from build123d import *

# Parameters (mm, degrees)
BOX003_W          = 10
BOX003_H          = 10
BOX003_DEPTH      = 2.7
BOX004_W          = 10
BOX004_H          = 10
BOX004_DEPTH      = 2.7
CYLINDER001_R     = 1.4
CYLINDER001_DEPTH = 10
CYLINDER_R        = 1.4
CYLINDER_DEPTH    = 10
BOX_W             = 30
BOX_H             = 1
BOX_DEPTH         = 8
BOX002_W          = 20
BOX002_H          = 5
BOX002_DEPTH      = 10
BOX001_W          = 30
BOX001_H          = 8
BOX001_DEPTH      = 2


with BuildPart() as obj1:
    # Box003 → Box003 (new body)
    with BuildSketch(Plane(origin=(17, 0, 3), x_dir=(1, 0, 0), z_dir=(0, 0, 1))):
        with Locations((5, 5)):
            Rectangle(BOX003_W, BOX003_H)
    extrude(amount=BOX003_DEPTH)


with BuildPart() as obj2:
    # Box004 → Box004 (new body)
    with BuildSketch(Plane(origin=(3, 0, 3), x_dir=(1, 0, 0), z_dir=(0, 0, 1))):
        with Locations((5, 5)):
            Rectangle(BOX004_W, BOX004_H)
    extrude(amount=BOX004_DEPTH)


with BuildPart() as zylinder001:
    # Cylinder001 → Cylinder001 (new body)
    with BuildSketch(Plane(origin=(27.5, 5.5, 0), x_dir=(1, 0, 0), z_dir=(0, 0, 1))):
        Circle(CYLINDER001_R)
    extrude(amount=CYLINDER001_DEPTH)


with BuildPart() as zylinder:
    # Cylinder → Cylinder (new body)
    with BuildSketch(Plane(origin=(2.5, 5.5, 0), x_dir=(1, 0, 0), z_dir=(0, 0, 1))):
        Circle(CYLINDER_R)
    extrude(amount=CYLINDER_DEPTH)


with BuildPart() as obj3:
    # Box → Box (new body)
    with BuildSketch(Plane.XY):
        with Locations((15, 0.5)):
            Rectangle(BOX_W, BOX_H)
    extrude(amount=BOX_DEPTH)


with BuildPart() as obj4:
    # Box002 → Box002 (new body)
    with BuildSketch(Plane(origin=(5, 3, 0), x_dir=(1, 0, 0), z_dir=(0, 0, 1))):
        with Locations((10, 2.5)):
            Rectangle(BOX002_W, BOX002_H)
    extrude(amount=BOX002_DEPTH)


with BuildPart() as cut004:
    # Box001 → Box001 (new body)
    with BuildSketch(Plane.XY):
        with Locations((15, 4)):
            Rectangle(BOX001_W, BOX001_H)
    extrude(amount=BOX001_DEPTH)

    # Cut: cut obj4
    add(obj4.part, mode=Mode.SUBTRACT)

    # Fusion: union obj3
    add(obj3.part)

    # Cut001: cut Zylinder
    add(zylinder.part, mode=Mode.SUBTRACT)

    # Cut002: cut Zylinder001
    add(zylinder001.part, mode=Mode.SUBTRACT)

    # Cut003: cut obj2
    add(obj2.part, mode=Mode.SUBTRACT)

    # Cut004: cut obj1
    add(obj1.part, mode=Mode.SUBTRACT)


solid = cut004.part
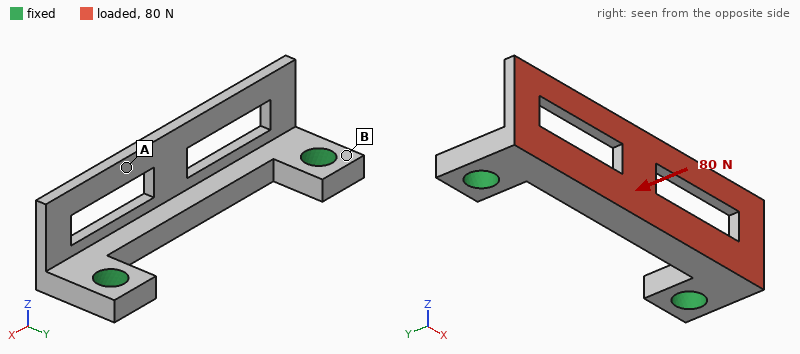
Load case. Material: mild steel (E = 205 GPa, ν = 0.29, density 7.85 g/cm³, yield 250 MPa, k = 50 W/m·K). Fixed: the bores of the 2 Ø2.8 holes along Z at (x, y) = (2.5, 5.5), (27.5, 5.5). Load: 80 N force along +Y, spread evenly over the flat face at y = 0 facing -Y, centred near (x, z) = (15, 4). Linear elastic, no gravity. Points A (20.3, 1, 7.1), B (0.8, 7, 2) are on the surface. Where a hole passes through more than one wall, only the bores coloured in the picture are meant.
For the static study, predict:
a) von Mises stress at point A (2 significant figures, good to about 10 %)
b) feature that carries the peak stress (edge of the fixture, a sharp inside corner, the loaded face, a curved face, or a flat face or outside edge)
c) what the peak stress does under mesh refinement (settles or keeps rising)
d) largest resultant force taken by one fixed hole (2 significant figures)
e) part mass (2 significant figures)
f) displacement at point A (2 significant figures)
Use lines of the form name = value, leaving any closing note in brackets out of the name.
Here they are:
von Mises stress at point A = 22 MPa
feature that carries the peak stress = a sharp inside corner
what the peak stress does under mesh refinement = keeps rising
largest resultant force taken by one fixed hole = 44 N
part mass = 3.0 g
displacement at point A = 20 µm
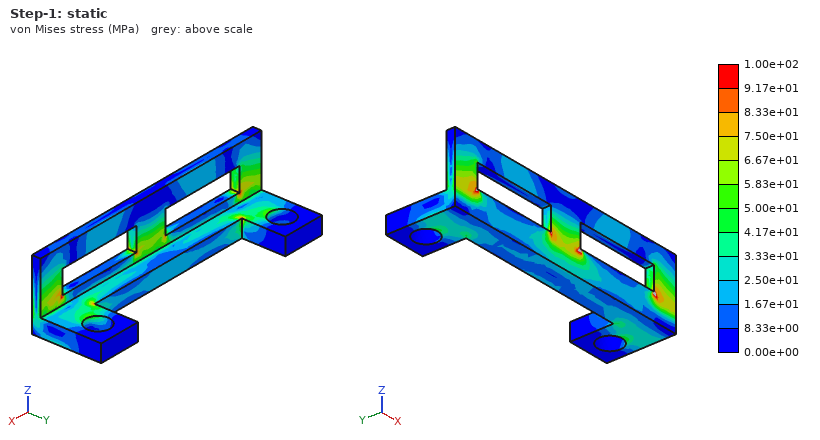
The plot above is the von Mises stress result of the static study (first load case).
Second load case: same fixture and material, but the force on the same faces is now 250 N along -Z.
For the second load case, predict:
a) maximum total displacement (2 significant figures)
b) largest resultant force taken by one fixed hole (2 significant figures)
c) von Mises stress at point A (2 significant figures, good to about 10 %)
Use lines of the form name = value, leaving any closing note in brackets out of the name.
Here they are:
maximum total displacement = 32 µm
largest resultant force taken by one fixed hole = 130 N
von Mises stress at point A = 32 MPa
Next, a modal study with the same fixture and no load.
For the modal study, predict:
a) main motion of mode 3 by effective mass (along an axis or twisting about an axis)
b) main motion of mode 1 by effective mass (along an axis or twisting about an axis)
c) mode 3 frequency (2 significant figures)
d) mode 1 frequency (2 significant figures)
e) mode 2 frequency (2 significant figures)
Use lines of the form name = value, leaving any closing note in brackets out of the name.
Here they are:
main motion of mode 3 by effective mass = along Z
main motion of mode 1 by effective mass = along Y
mode 3 frequency = 17 kHz
mode 1 frequency = 9300 Hz
mode 2 frequency = 14 kHz
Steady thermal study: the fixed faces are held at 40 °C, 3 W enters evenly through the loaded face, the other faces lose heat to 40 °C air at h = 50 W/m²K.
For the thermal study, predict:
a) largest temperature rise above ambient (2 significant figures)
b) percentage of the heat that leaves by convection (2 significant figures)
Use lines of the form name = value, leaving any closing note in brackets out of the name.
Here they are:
largest temperature rise above ambient = 30 K
percentage of the heat that leaves by convection = 13 %
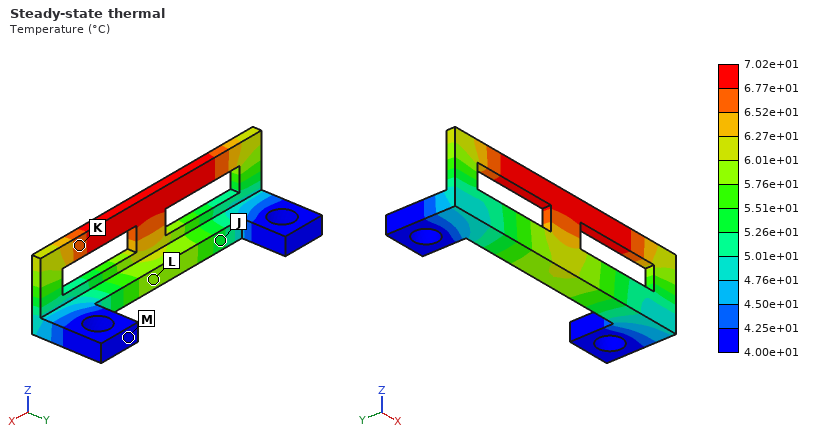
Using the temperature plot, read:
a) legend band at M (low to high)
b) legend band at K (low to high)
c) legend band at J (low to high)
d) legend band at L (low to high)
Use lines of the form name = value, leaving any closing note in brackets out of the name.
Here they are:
legend band at M = 4.00e+01 to 4.25e+01 °C
legend band at K = 6.52e+01 to 6.77e+01 °C
legend band at J = 5.26e+01 to 5.51e+01 °C
legend band at L = 5.76e+01 to 6.01e+01 °C
